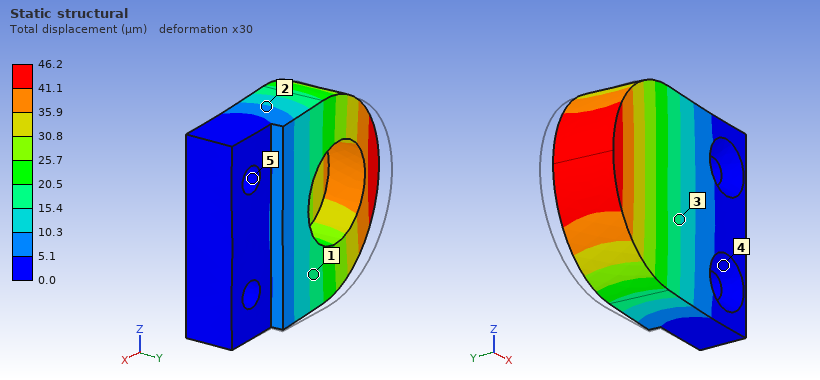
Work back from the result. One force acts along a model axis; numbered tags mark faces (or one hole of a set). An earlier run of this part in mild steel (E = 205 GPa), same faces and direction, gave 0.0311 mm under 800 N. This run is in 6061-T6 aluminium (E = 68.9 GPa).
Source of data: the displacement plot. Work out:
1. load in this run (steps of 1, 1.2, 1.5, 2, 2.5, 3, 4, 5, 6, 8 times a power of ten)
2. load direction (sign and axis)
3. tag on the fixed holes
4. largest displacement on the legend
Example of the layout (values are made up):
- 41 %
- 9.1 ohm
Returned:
- 400 N
- -Y
- 5
- 46.2 µm
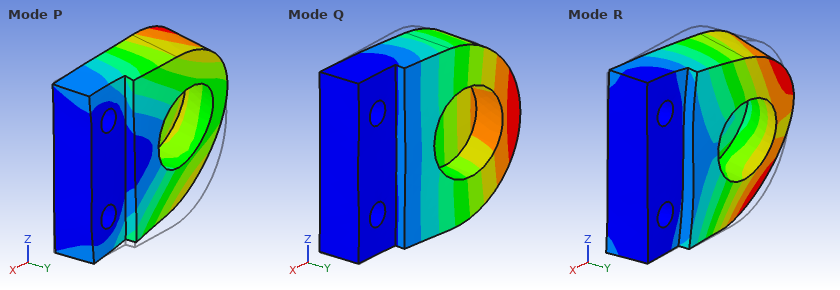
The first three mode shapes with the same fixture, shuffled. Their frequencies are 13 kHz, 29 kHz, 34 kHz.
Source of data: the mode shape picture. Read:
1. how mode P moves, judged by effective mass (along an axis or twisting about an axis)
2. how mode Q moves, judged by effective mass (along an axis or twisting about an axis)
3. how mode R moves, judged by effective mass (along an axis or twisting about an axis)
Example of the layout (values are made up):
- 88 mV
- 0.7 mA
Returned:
- along Z
- along Y
- along Z
